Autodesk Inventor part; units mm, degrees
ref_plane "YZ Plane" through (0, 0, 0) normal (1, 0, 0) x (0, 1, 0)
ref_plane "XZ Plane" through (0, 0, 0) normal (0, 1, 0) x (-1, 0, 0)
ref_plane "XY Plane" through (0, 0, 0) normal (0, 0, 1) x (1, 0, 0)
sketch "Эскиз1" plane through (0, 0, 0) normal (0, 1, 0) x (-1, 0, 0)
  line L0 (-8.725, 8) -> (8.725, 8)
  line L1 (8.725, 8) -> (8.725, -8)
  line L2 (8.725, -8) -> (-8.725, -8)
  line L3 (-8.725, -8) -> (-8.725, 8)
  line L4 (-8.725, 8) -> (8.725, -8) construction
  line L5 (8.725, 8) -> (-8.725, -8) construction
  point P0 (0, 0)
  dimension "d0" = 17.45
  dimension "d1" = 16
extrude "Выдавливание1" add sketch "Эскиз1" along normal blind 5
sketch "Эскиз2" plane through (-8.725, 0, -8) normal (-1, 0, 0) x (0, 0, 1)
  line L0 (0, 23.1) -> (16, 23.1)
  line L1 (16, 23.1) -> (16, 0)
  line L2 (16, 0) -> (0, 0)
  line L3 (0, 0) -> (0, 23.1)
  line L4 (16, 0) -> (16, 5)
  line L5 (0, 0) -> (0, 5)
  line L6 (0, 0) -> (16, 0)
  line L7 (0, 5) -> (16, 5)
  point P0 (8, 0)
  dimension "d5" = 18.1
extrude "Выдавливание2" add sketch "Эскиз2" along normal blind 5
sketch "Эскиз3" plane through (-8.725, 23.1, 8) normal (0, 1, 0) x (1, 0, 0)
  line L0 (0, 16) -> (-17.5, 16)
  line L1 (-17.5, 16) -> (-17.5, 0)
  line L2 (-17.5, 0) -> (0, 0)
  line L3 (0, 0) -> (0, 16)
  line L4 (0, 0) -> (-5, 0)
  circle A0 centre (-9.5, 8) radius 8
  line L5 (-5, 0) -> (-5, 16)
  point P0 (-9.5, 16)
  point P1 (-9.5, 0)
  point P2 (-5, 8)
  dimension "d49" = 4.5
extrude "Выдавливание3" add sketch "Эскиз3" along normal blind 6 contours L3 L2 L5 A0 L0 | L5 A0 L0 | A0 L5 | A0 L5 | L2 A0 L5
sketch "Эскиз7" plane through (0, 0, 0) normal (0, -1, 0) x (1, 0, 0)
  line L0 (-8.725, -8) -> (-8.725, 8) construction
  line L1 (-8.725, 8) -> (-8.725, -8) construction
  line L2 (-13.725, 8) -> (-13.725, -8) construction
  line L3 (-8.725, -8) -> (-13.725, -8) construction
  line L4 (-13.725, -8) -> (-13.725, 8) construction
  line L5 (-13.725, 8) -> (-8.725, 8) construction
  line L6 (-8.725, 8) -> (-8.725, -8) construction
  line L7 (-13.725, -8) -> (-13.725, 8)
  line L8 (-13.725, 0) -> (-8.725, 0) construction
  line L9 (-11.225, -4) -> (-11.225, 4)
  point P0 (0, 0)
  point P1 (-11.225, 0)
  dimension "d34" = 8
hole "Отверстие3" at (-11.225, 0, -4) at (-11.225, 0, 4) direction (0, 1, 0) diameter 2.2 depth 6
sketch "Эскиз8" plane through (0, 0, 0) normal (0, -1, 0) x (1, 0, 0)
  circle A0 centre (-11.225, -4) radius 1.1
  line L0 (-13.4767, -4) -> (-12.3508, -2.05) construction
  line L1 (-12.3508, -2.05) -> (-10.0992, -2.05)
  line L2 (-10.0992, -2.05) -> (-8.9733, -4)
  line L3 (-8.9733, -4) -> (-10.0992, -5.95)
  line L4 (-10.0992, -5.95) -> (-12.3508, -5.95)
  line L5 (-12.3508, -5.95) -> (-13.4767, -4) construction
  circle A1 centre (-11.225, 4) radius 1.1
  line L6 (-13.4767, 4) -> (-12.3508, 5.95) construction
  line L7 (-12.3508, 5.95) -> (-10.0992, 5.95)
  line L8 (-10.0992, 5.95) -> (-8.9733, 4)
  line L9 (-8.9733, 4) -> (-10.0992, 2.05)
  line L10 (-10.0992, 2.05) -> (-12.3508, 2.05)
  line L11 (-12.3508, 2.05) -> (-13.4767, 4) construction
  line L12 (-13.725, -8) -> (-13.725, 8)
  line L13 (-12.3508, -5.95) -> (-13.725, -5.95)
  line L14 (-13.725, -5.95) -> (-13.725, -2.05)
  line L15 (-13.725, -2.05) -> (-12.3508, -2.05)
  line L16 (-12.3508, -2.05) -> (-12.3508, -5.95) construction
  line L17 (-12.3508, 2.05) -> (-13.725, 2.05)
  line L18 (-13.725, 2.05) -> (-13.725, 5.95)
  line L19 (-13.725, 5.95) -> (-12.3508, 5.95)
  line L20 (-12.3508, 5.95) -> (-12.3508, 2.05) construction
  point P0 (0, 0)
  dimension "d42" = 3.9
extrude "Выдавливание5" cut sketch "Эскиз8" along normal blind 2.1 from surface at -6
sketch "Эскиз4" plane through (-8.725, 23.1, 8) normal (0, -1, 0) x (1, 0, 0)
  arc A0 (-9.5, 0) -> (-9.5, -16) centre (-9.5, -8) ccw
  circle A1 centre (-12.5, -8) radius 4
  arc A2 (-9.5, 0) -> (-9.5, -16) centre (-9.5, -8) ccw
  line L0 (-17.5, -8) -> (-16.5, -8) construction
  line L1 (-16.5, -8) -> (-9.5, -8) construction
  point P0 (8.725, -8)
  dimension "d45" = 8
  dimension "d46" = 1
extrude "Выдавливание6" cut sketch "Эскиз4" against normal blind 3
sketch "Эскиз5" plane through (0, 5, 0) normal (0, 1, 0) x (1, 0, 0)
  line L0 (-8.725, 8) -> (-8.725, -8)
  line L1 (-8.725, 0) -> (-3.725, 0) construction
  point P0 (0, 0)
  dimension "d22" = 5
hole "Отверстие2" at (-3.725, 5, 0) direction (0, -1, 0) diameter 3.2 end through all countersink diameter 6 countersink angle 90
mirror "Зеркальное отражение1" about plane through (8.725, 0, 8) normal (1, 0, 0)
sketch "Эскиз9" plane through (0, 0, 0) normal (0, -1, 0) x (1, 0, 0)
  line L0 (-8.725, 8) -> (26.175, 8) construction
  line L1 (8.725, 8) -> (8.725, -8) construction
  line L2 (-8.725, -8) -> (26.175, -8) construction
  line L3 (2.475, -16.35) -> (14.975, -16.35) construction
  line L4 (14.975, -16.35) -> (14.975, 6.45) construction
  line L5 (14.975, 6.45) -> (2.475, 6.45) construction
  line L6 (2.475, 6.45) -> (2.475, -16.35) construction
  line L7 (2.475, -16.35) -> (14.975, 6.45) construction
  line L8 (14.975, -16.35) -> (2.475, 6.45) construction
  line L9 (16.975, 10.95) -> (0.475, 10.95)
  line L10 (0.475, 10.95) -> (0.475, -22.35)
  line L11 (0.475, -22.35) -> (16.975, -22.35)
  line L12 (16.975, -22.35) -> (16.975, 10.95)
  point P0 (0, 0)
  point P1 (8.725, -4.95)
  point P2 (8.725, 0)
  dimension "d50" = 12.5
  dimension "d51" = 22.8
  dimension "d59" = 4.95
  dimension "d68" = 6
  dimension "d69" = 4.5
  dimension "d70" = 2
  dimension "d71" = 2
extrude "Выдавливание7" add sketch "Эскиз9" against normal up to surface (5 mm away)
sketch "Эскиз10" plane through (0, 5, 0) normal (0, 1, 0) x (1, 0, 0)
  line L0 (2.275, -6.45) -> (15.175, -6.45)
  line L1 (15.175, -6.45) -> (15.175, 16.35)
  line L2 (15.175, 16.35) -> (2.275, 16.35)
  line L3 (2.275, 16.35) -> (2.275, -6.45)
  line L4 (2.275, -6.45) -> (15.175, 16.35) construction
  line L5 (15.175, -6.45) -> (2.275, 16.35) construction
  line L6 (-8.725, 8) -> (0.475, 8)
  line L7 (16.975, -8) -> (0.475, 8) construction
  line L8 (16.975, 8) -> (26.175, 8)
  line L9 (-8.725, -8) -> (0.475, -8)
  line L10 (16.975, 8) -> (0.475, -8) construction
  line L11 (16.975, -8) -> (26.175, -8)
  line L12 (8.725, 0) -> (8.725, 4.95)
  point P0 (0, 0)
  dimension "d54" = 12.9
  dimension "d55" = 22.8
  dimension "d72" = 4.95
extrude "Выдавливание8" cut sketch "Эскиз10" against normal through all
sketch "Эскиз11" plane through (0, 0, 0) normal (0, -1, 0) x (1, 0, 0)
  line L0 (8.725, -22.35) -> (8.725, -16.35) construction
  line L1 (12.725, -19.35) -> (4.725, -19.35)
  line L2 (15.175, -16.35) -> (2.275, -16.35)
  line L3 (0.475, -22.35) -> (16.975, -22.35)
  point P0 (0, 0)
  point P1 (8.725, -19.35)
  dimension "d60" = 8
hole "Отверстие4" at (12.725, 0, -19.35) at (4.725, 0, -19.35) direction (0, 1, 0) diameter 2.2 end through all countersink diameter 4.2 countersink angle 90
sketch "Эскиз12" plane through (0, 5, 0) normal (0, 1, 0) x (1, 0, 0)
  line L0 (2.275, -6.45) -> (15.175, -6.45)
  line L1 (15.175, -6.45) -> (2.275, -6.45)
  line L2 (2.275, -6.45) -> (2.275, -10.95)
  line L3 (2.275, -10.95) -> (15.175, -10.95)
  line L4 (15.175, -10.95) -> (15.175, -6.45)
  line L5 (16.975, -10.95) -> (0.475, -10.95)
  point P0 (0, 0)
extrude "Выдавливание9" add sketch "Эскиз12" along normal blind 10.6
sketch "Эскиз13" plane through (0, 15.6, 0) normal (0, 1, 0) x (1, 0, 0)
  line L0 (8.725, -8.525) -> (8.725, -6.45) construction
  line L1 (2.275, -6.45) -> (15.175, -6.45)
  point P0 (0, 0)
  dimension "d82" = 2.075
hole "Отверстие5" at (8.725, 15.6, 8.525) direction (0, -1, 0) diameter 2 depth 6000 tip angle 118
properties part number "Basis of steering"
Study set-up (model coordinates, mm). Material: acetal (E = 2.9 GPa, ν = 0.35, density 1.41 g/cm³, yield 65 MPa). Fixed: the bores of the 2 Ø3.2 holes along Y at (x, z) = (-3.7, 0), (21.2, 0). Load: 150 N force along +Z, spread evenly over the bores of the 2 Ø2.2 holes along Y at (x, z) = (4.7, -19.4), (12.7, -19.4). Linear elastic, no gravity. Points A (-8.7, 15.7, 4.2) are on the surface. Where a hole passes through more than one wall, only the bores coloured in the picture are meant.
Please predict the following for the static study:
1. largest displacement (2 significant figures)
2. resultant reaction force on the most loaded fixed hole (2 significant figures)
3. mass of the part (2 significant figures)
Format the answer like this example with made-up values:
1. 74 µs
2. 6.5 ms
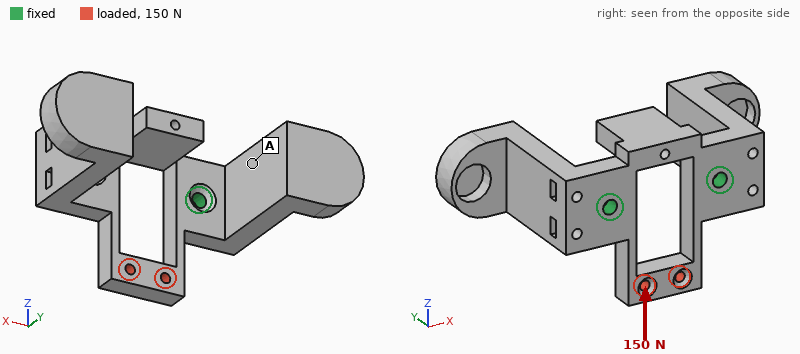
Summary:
1. 0.16 mm
2. 76 N
3. 13 g
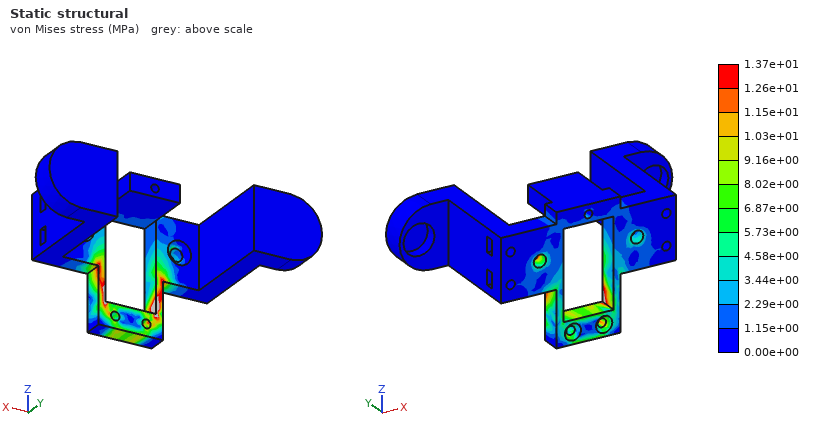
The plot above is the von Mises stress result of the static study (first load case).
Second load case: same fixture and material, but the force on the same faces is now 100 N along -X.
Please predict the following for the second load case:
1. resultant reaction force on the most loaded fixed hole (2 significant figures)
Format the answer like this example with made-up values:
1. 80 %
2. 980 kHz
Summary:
1. 72 N
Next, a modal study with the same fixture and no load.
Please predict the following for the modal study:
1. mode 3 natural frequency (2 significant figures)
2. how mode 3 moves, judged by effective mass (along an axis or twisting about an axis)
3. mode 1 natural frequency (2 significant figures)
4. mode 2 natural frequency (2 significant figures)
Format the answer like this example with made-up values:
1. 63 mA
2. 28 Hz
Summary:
1. 970 Hz
2. along Z
3. 650 Hz
4. 650 Hz
